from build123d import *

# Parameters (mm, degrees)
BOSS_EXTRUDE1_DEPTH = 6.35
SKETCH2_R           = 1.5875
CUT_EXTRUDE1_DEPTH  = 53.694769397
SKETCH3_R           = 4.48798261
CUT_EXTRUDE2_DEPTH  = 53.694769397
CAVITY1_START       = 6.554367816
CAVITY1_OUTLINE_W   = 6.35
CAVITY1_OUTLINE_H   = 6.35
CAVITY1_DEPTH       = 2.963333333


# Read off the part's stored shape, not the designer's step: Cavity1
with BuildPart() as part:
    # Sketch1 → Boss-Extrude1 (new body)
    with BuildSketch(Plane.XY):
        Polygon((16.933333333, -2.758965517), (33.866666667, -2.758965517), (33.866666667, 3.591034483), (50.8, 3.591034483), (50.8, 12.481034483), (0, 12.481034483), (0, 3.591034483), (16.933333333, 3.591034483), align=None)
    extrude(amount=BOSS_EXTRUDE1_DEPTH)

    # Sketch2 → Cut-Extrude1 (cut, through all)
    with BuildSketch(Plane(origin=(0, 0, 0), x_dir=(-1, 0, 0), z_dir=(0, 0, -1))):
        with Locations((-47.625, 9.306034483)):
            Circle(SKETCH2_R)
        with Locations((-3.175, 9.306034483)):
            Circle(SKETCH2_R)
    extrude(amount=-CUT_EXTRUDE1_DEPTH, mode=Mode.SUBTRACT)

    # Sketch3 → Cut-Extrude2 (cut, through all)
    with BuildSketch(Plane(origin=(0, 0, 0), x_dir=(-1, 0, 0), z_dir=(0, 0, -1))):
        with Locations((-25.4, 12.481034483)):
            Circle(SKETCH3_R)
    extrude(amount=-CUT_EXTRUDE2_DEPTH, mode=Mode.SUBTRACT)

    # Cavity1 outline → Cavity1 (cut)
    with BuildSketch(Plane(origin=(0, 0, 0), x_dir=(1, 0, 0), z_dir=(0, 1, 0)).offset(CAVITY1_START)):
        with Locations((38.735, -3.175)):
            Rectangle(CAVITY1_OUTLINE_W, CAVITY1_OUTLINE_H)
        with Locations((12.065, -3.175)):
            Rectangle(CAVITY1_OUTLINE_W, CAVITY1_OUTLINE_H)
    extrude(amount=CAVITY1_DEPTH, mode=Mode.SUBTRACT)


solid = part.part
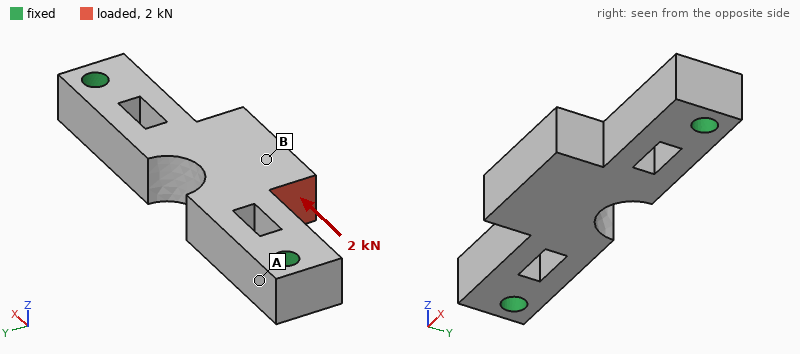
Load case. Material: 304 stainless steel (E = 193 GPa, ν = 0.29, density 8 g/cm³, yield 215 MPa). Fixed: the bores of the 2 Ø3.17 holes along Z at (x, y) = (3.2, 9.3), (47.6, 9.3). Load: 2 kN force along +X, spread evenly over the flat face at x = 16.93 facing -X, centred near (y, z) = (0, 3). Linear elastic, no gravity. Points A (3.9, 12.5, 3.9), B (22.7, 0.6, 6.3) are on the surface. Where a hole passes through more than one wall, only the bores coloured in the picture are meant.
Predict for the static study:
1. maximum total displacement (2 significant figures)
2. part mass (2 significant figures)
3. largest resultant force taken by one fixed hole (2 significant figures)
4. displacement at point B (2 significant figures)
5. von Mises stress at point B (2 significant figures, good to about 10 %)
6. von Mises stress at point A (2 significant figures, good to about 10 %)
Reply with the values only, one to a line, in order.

11 µm
24 g
1.1 kN
6.6 µm
33 MPa
15 MPa
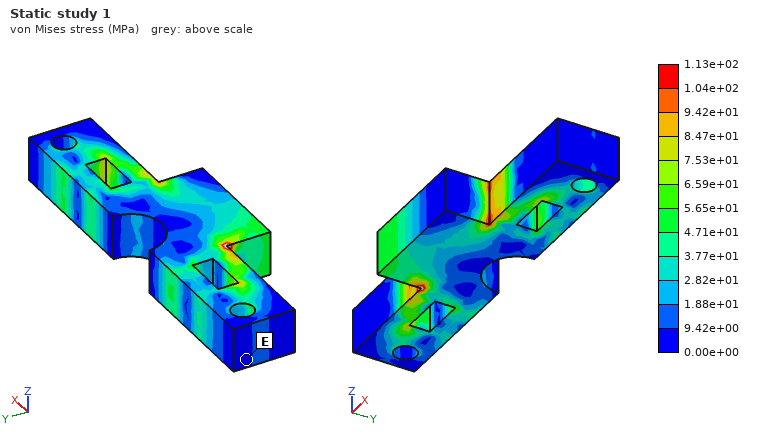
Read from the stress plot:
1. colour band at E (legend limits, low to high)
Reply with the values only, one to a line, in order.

0.00e+00 to 9.42e+00 MPa
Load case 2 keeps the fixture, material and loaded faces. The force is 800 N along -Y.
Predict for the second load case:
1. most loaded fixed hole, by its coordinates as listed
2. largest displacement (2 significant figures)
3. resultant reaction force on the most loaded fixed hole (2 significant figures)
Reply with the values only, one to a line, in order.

(3.2, 9.3)
15 µm
670 N
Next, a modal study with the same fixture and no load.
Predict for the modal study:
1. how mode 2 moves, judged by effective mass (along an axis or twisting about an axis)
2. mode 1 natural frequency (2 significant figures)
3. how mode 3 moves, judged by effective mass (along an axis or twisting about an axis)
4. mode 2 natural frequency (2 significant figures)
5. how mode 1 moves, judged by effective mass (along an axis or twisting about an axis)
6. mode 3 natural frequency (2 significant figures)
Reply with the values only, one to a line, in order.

along Y
9400 Hz
along Z
12 kHz
along Z
19 kHz
